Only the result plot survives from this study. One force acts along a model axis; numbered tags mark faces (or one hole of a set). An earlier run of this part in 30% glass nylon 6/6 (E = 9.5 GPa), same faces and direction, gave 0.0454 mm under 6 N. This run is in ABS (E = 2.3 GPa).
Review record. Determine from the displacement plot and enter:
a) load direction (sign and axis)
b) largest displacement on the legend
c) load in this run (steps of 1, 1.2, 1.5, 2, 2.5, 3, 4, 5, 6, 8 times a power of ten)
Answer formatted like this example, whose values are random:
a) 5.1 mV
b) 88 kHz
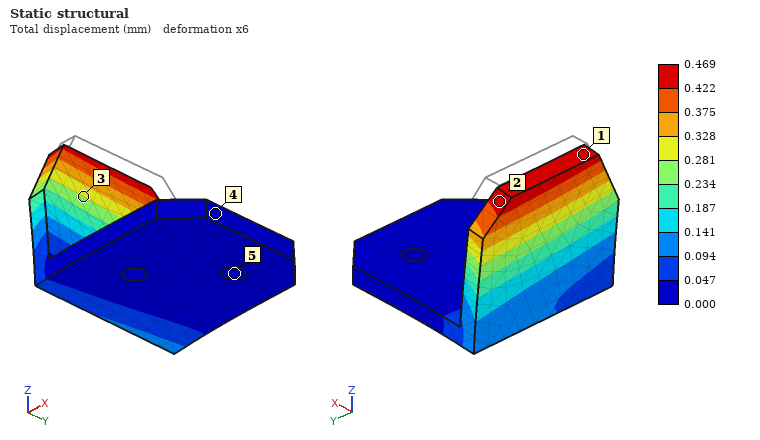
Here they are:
a) -X
b) 0.469 mm
c) 15 N
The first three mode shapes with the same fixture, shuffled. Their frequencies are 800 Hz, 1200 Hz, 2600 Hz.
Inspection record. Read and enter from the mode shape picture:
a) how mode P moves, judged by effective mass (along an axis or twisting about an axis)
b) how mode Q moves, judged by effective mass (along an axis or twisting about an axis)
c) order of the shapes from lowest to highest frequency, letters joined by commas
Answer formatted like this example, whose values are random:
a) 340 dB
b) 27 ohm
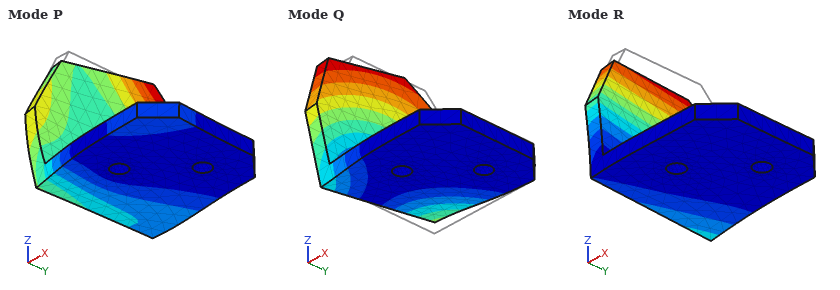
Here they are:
a) along Z
b) along Y
c) R, Q, P
